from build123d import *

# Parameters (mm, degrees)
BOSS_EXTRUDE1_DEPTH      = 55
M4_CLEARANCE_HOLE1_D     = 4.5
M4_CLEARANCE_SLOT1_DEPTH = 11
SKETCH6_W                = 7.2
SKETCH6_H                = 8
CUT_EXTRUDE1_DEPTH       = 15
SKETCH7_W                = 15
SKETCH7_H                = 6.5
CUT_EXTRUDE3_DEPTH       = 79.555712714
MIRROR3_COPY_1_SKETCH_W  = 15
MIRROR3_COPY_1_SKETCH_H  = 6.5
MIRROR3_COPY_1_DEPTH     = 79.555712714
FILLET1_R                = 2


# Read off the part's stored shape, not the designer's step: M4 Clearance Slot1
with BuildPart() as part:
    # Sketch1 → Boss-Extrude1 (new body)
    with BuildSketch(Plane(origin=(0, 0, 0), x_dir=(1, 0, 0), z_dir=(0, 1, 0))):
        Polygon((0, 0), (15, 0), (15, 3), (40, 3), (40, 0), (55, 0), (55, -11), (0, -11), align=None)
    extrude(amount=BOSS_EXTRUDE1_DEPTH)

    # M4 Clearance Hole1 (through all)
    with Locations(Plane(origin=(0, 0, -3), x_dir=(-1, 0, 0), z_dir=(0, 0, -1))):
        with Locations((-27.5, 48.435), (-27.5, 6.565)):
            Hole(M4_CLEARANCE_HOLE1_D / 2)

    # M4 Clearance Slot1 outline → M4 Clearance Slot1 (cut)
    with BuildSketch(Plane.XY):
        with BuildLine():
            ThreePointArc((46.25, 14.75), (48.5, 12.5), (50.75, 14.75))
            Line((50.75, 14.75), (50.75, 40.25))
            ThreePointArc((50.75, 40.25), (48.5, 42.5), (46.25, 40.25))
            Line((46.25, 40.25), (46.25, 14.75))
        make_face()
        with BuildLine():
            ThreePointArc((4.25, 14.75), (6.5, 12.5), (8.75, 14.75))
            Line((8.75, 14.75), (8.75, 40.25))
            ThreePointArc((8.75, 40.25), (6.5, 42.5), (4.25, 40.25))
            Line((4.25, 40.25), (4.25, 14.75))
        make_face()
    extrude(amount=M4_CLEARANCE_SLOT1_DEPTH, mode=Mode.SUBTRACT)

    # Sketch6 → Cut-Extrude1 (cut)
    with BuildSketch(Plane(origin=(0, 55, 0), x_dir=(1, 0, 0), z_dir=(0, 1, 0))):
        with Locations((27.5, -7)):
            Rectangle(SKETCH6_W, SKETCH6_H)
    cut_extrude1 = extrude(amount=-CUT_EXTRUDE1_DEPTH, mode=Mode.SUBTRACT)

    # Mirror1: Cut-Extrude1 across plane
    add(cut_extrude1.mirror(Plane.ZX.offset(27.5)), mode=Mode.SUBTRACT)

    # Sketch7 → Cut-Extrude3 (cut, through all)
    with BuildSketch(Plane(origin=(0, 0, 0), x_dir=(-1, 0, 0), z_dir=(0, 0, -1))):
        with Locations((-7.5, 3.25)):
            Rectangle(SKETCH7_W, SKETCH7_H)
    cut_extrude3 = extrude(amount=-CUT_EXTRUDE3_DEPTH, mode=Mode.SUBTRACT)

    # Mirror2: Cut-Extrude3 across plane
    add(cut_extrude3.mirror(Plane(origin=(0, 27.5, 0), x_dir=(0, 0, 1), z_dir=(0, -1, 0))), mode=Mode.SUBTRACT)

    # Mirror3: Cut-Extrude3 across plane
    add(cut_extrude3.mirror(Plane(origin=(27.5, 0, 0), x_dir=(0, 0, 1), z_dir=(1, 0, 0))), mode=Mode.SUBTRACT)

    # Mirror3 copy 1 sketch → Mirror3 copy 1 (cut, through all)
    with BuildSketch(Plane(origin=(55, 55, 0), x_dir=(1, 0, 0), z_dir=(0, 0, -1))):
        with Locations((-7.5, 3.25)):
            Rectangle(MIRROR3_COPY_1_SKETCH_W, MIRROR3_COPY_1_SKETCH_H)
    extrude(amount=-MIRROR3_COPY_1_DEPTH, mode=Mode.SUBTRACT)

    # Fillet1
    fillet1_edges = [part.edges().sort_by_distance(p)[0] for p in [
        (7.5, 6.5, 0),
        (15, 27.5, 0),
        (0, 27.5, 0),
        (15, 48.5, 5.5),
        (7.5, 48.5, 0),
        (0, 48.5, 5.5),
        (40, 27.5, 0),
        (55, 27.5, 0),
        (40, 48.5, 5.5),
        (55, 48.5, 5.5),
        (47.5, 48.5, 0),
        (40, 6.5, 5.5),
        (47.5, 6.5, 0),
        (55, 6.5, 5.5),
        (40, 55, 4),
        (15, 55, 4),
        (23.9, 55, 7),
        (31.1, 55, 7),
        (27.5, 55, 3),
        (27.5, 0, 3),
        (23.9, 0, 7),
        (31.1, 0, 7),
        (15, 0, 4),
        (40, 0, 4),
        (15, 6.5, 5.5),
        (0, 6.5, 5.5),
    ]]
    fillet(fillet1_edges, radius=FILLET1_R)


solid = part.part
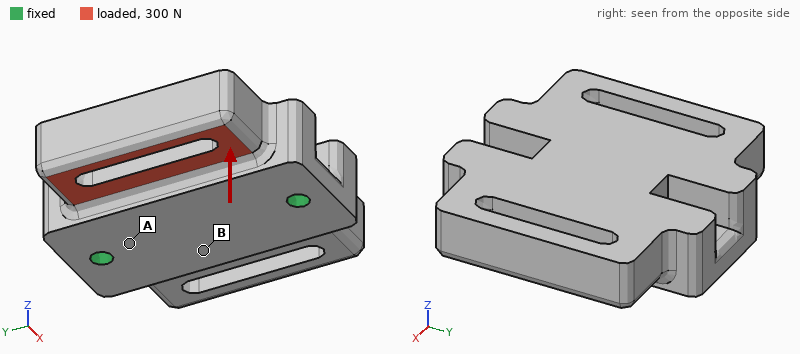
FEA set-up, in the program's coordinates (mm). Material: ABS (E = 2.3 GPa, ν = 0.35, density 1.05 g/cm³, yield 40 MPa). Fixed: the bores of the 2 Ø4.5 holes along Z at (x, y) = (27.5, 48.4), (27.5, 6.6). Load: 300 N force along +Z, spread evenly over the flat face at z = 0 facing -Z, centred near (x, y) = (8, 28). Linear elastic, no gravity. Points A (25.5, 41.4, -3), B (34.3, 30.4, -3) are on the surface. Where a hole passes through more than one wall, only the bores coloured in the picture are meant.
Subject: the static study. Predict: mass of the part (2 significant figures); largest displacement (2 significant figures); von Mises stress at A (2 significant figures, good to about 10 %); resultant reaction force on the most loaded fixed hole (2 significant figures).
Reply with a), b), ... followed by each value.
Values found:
a) 30 g
b) 0.48 mm
c) 4.8 MPa
d) 180 N
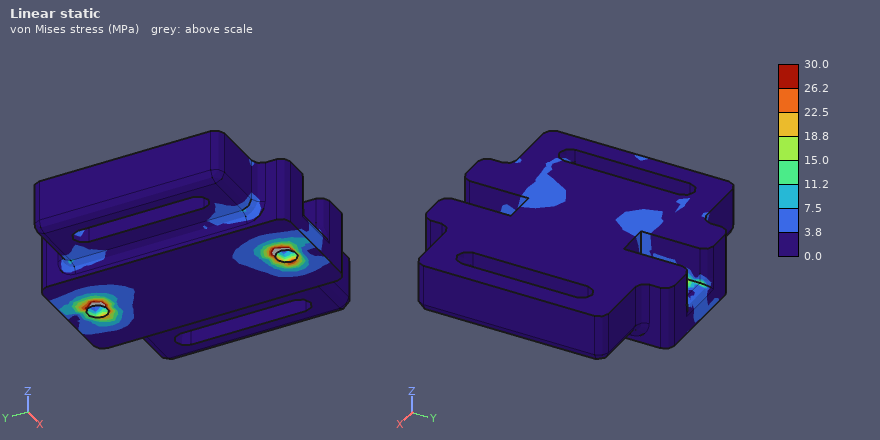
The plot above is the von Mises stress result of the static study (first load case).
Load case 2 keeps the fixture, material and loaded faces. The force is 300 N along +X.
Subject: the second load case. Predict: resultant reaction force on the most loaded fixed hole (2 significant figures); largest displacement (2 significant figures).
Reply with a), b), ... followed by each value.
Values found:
a) 150 N
b) 0.14 mm
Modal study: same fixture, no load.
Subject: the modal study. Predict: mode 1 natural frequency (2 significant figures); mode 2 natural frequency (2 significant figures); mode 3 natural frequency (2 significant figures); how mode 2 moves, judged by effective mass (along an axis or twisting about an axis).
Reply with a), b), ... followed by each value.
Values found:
a) 1400 Hz
b) 2900 Hz
c) 4200 Hz
d) along Z
